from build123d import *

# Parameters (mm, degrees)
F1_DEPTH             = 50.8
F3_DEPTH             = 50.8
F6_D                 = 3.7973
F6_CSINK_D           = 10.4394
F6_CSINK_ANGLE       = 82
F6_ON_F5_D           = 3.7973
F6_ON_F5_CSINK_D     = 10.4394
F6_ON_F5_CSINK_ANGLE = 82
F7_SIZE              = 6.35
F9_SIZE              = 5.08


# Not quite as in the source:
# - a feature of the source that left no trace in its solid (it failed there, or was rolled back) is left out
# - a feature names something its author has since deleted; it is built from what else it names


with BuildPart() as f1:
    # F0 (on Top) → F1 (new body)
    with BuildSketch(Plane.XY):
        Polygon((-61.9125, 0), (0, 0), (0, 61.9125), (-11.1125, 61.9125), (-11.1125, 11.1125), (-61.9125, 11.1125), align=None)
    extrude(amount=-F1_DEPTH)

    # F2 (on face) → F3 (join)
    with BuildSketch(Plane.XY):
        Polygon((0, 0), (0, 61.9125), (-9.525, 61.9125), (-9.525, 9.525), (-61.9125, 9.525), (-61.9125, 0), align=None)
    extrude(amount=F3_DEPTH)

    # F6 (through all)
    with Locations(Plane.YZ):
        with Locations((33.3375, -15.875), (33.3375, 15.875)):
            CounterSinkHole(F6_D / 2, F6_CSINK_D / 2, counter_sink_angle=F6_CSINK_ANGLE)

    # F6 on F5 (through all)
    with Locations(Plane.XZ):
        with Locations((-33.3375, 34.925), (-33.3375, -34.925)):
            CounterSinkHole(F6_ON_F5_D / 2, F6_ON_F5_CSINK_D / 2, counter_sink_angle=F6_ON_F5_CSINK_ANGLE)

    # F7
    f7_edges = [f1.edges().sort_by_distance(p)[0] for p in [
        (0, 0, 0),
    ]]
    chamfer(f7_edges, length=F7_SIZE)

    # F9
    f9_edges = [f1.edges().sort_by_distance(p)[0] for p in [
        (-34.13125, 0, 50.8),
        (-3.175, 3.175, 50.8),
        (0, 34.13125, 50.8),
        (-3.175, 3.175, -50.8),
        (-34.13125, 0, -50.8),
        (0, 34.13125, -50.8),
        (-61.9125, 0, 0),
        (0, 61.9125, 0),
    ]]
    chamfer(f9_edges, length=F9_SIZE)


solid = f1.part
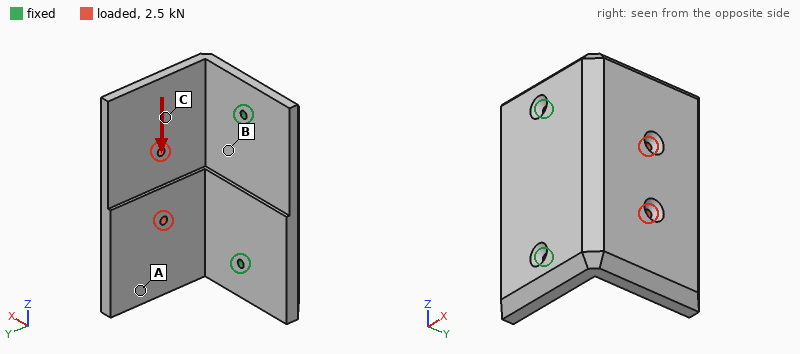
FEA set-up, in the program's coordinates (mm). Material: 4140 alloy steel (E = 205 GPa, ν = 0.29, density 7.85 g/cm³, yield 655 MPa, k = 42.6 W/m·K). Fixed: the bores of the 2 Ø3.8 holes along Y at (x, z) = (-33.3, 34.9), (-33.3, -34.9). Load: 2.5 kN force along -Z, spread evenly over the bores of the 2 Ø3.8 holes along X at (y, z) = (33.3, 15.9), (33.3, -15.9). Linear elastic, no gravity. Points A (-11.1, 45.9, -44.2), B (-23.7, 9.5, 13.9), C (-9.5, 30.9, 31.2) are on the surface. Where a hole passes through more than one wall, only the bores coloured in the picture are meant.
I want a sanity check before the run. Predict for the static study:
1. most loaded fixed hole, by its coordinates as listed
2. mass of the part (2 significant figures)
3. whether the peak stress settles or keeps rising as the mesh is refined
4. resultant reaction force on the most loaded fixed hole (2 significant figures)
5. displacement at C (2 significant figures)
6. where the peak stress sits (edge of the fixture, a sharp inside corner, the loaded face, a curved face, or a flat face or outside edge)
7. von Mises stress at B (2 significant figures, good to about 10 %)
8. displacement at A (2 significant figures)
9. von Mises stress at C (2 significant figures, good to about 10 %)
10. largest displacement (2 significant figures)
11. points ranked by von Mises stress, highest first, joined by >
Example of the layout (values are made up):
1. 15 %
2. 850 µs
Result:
1. (-33.3, -34.9)
2. 870 g
3. keeps rising
4. 2.0 kN
5. 16 µm
6. edge of the fixture
7. 19 MPa
8. 20 µm
9. 9.5 MPa
10. 29 µm
11. B > C > A
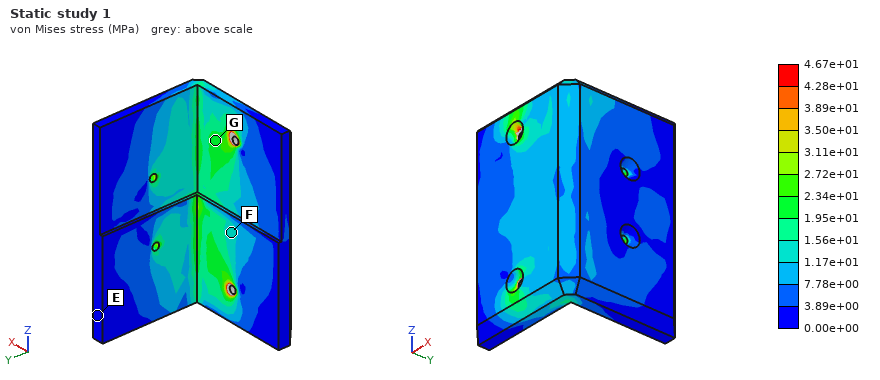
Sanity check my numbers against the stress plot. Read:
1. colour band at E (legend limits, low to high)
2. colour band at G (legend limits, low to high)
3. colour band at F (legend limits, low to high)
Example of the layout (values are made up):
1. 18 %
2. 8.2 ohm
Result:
1. 0.00e+00 to 3.89e+00 MPa
2. 1.95e+01 to 2.34e+01 MPa
3. 1.17e+01 to 1.56e+01 MPa
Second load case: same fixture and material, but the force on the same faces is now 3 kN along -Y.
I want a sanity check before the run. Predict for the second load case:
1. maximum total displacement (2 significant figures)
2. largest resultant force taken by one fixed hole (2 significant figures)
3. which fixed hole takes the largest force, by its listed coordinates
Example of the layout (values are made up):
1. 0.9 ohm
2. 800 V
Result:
1. 0.11 mm
2. 1.6 kN
3. (-33.3, -34.9)
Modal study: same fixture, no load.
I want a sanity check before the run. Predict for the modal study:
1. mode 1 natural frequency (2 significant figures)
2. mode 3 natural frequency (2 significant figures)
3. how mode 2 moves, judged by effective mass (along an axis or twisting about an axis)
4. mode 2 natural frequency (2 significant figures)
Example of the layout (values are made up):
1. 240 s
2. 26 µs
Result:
1. 1100 Hz
2. 3400 Hz
3. along Z
4. 2400 Hz
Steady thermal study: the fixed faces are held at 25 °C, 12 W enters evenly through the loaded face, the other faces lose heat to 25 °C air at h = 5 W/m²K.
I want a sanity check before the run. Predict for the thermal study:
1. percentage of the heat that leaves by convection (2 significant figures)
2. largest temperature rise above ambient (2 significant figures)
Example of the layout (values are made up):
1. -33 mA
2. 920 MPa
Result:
1. 11 %
2. 23 K
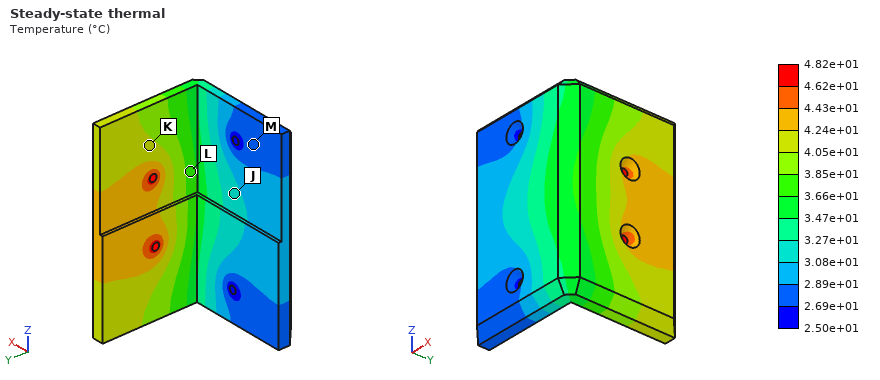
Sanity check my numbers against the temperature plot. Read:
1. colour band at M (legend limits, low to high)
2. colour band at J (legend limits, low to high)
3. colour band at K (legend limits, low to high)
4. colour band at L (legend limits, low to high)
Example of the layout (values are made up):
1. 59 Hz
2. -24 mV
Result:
1. 2.69e+01 to 2.89e+01 °C
2. 3.08e+01 to 3.27e+01 °C
3. 4.05e+01 to 4.24e+01 °C
4. 3.66e+01 to 3.85e+01 °C
